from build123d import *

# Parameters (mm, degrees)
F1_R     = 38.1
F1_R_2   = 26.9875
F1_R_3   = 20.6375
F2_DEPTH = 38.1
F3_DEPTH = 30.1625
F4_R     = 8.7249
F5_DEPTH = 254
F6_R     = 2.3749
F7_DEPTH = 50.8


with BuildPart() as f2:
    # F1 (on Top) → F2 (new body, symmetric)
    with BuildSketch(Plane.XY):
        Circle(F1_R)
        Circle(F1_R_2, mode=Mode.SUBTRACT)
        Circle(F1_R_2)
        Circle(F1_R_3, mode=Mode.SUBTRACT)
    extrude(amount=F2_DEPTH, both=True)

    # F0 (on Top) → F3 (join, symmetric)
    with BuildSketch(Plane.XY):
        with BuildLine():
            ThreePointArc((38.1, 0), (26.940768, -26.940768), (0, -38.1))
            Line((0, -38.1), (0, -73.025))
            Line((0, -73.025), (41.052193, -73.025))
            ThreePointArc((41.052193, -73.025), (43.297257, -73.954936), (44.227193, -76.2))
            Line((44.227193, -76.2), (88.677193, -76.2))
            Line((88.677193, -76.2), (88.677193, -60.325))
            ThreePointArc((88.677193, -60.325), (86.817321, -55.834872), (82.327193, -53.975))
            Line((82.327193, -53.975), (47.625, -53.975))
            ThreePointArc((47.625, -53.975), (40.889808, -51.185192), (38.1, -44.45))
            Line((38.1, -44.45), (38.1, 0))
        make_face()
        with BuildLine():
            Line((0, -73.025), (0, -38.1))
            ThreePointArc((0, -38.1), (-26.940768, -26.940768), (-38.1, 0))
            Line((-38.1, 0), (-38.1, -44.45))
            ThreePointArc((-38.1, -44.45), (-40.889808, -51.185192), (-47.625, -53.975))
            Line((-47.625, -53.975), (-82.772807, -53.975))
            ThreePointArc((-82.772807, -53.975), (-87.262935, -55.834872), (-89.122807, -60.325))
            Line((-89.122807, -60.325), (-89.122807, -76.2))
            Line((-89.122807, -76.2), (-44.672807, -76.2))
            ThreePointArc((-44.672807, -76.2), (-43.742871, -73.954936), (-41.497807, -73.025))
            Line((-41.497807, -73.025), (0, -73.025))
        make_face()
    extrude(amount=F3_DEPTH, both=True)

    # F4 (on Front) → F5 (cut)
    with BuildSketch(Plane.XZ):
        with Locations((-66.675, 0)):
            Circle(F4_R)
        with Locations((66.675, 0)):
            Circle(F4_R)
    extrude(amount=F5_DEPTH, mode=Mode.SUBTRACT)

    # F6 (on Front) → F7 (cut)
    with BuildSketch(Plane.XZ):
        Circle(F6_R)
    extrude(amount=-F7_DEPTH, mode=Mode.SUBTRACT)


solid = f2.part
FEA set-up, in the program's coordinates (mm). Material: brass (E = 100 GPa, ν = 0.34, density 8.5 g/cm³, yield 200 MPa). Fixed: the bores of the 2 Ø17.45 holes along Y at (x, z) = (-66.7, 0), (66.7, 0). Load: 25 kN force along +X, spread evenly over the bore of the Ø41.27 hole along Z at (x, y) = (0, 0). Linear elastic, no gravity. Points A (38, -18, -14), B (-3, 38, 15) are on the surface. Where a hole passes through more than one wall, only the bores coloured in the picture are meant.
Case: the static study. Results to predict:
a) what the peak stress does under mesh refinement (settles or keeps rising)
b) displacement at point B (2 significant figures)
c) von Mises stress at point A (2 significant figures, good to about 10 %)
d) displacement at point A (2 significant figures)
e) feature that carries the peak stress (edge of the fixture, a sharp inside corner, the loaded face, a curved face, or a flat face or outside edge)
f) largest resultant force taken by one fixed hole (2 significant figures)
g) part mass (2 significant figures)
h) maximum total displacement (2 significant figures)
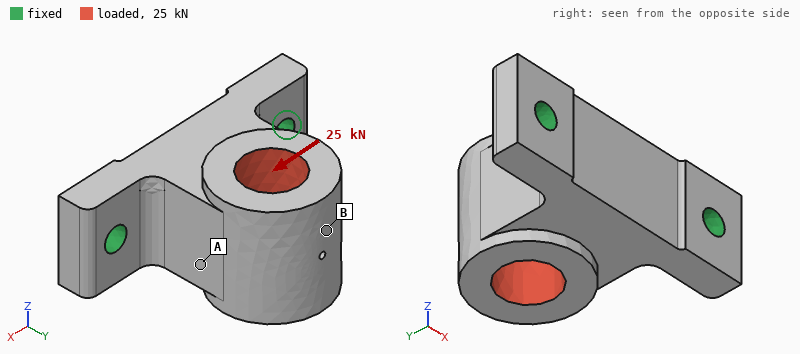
keeps rising
75 µm
18 MPa
37 µm
edge of the fixture
20 kN
4.8 kg
75 µm
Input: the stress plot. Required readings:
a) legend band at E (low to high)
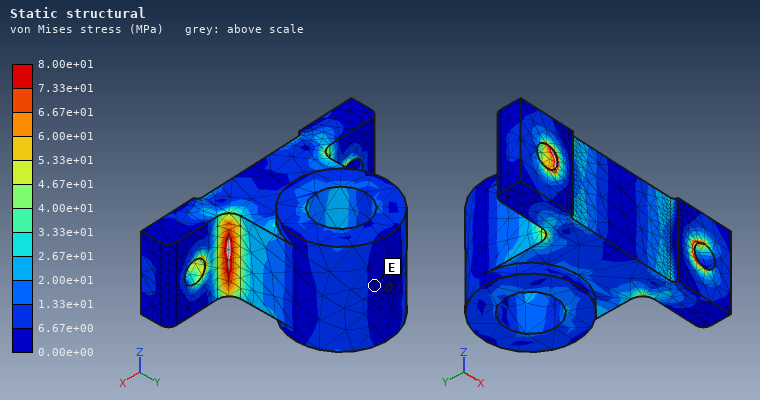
0.00e+00 to 6.67e+00 MPa
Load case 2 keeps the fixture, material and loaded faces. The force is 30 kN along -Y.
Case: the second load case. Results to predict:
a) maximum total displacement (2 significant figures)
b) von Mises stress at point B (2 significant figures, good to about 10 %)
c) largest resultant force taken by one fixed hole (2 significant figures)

30 µm
6.4 MPa
17 kN
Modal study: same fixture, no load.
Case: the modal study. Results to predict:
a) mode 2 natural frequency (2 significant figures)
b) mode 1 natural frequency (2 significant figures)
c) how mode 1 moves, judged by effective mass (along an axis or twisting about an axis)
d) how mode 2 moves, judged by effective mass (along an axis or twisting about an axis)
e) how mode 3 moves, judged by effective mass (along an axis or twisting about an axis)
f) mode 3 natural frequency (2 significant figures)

2200 Hz
940 Hz
along Z
along X
along Y
2800 Hz
